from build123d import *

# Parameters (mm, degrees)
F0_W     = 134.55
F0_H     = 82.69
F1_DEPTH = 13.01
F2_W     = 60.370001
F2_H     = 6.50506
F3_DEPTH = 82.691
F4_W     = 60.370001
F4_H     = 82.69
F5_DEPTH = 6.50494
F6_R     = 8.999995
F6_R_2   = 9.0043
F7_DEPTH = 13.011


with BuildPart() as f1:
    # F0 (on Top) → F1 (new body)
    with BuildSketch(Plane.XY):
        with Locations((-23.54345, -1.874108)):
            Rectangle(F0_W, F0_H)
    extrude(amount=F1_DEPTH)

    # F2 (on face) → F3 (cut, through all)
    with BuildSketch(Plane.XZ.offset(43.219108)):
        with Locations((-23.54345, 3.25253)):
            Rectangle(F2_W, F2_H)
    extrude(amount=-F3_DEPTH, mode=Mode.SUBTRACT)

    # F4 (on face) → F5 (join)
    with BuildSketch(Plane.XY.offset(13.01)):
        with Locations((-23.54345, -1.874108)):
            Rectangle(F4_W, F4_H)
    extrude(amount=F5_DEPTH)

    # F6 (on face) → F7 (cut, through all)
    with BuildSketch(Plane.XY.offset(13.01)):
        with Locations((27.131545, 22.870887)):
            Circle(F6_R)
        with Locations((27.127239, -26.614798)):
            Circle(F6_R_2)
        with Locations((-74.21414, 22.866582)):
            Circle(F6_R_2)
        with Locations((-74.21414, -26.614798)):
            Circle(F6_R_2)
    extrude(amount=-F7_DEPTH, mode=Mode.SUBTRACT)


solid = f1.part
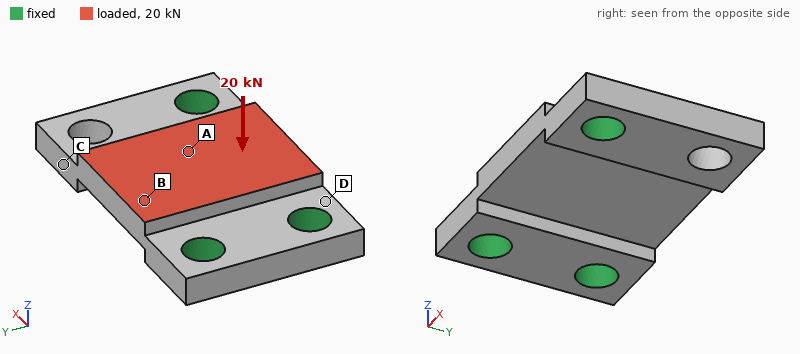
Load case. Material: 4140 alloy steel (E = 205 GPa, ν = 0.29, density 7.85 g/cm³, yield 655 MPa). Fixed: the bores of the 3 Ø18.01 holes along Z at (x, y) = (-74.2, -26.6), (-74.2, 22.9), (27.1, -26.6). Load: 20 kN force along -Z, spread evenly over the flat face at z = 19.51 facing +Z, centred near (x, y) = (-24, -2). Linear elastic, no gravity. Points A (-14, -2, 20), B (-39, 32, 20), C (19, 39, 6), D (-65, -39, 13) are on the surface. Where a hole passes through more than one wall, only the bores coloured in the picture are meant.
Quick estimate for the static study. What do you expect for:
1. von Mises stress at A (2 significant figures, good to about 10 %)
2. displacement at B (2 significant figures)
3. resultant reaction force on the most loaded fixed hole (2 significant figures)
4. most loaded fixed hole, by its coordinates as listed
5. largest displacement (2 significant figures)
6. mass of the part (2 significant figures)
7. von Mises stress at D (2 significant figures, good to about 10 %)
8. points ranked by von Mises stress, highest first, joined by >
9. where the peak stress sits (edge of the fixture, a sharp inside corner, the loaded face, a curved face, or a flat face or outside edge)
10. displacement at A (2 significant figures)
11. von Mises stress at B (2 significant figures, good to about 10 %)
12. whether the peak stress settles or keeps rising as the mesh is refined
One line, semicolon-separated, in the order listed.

62 MPa; 33 µm; 15 kN; (27.1, -26.6); 69 µm; 1.0 kg; 22 MPa; A > B > D > C; edge of the fixture; 32 µm; 45 MPa; keeps rising
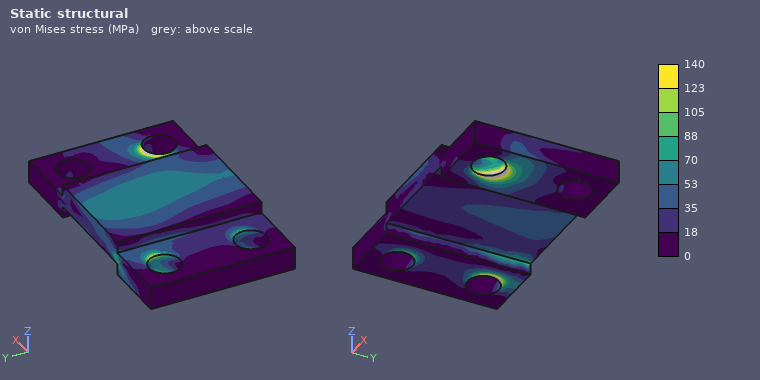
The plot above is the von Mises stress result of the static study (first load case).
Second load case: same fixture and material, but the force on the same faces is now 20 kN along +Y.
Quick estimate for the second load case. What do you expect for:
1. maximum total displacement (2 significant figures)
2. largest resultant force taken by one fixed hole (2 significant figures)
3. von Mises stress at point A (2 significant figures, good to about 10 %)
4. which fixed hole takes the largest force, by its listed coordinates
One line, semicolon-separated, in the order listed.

37 µm; 9.7 kN; 13 MPa; (-74.2, -26.6)
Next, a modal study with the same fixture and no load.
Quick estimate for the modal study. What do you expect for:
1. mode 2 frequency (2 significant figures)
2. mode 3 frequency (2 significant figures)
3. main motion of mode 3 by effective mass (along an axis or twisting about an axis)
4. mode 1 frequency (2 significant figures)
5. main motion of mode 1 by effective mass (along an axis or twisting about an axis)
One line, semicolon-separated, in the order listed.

6400 Hz; 8600 Hz; along Z; 3600 Hz; along Z
